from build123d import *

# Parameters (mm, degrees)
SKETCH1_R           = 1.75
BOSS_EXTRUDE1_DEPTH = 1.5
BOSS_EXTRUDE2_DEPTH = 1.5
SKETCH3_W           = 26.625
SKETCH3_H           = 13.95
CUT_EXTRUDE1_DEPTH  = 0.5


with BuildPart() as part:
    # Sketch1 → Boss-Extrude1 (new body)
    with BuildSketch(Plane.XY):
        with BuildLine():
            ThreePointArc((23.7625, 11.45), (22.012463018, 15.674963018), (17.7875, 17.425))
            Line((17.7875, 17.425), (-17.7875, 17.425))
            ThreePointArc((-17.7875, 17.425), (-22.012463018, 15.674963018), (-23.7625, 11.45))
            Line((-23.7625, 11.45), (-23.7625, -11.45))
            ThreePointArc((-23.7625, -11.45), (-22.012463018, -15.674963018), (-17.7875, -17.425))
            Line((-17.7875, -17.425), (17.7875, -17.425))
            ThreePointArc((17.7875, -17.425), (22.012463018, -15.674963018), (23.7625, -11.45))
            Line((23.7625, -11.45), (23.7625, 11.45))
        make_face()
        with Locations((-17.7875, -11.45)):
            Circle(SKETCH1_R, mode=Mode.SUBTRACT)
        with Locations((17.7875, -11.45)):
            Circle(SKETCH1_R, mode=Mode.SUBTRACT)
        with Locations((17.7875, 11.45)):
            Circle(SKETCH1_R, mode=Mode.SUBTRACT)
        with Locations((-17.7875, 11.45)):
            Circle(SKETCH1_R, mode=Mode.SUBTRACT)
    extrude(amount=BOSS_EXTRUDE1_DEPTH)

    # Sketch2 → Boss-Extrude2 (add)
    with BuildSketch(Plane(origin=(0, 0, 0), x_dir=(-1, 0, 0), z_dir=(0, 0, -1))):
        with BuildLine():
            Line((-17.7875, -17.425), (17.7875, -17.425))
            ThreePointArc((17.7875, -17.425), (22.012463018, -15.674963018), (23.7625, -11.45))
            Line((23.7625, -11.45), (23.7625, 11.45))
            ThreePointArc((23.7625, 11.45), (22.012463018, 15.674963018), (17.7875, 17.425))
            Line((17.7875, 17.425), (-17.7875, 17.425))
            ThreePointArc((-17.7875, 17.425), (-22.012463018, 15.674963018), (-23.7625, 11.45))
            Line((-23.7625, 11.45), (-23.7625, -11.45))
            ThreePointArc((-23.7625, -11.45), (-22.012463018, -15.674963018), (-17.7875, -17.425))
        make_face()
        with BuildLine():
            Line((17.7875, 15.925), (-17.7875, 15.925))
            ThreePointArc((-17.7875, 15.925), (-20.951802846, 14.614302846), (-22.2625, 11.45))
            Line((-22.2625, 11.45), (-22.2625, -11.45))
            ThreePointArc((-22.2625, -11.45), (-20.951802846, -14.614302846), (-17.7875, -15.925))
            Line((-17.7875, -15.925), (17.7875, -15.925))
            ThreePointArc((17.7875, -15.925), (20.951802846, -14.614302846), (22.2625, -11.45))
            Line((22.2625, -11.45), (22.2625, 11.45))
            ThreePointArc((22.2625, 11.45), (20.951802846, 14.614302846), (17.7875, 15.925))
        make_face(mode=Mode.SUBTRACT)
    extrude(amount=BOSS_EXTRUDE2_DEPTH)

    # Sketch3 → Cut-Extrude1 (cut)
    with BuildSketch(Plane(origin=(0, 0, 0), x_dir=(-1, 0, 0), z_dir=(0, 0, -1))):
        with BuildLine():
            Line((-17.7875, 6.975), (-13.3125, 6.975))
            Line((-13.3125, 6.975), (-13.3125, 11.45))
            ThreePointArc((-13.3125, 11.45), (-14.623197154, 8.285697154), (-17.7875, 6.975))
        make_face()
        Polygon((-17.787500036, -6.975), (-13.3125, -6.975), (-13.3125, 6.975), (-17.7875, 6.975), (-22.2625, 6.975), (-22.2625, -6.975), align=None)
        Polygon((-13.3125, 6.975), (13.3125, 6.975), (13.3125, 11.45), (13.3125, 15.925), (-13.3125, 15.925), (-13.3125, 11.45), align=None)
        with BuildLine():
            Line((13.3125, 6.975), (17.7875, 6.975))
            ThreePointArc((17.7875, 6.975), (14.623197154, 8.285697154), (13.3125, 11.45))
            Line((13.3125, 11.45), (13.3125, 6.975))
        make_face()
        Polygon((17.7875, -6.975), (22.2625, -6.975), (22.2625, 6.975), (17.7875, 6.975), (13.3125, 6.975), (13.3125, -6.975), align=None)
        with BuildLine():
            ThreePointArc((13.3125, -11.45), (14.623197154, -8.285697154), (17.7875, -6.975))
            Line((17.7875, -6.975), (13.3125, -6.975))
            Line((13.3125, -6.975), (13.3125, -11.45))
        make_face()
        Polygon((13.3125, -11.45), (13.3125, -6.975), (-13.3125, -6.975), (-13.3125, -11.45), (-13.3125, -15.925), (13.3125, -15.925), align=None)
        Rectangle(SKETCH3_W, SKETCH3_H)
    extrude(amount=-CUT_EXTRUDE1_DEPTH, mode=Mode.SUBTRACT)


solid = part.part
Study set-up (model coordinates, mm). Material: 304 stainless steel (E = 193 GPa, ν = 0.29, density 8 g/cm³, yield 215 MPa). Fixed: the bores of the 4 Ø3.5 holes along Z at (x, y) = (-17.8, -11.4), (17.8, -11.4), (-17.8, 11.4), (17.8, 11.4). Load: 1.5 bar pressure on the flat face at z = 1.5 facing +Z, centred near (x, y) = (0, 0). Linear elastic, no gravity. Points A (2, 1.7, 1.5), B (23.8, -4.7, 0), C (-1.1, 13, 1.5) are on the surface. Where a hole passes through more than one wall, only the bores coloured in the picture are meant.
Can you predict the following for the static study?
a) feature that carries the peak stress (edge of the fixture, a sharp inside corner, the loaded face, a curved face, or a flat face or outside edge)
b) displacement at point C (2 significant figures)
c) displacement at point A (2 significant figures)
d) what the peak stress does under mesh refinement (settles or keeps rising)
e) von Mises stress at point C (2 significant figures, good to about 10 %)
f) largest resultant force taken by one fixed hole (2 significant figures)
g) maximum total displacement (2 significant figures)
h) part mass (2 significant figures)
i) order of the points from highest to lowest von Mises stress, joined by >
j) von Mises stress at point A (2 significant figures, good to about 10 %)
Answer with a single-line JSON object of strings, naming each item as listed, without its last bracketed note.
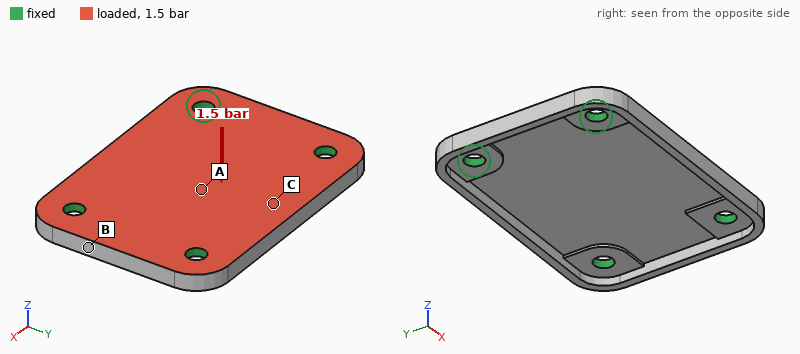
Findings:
{"feature that carries the peak stress": "edge of the fixture", "displacement at point C": "11 µm", "displacement at point A": "21 µm", "what the peak stress does under mesh refinement": "keeps rising", "von Mises stress at point C": "17 MPa", "largest resultant force taken by one fixed hole": "69 N", "maximum total displacement": "22 µm", "part mass": "17 g", "order of the points from highest to lowest von Mises stress, joined by >": "A > C > B", "von Mises stress at point A": "28 MPa"}
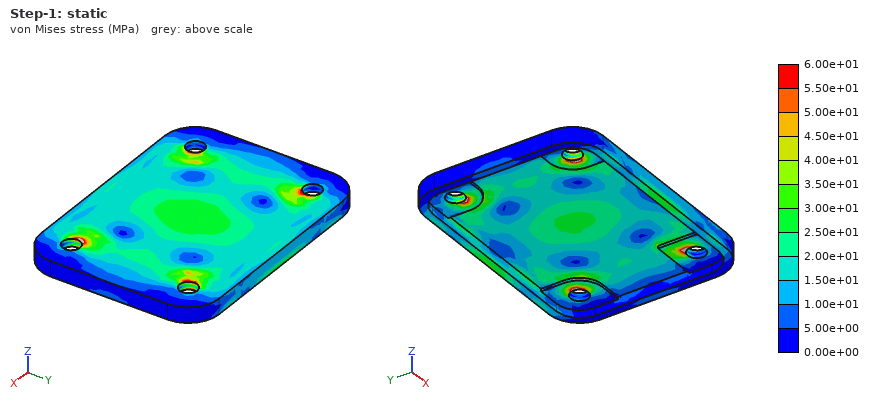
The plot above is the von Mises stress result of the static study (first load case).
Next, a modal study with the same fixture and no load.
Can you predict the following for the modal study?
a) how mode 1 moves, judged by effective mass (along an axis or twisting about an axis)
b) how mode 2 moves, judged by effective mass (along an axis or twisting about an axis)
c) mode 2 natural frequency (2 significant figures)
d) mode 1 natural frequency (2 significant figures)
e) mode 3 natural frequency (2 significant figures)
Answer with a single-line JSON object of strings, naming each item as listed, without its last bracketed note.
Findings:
{"how mode 1 moves, judged by effective mass": "along Z", "how mode 2 moves, judged by effective mass": "twisting about X", "mode 2 natural frequency": "8700 Hz", "mode 1 natural frequency": "5800 Hz", "mode 3 natural frequency": "10 kHz"}
